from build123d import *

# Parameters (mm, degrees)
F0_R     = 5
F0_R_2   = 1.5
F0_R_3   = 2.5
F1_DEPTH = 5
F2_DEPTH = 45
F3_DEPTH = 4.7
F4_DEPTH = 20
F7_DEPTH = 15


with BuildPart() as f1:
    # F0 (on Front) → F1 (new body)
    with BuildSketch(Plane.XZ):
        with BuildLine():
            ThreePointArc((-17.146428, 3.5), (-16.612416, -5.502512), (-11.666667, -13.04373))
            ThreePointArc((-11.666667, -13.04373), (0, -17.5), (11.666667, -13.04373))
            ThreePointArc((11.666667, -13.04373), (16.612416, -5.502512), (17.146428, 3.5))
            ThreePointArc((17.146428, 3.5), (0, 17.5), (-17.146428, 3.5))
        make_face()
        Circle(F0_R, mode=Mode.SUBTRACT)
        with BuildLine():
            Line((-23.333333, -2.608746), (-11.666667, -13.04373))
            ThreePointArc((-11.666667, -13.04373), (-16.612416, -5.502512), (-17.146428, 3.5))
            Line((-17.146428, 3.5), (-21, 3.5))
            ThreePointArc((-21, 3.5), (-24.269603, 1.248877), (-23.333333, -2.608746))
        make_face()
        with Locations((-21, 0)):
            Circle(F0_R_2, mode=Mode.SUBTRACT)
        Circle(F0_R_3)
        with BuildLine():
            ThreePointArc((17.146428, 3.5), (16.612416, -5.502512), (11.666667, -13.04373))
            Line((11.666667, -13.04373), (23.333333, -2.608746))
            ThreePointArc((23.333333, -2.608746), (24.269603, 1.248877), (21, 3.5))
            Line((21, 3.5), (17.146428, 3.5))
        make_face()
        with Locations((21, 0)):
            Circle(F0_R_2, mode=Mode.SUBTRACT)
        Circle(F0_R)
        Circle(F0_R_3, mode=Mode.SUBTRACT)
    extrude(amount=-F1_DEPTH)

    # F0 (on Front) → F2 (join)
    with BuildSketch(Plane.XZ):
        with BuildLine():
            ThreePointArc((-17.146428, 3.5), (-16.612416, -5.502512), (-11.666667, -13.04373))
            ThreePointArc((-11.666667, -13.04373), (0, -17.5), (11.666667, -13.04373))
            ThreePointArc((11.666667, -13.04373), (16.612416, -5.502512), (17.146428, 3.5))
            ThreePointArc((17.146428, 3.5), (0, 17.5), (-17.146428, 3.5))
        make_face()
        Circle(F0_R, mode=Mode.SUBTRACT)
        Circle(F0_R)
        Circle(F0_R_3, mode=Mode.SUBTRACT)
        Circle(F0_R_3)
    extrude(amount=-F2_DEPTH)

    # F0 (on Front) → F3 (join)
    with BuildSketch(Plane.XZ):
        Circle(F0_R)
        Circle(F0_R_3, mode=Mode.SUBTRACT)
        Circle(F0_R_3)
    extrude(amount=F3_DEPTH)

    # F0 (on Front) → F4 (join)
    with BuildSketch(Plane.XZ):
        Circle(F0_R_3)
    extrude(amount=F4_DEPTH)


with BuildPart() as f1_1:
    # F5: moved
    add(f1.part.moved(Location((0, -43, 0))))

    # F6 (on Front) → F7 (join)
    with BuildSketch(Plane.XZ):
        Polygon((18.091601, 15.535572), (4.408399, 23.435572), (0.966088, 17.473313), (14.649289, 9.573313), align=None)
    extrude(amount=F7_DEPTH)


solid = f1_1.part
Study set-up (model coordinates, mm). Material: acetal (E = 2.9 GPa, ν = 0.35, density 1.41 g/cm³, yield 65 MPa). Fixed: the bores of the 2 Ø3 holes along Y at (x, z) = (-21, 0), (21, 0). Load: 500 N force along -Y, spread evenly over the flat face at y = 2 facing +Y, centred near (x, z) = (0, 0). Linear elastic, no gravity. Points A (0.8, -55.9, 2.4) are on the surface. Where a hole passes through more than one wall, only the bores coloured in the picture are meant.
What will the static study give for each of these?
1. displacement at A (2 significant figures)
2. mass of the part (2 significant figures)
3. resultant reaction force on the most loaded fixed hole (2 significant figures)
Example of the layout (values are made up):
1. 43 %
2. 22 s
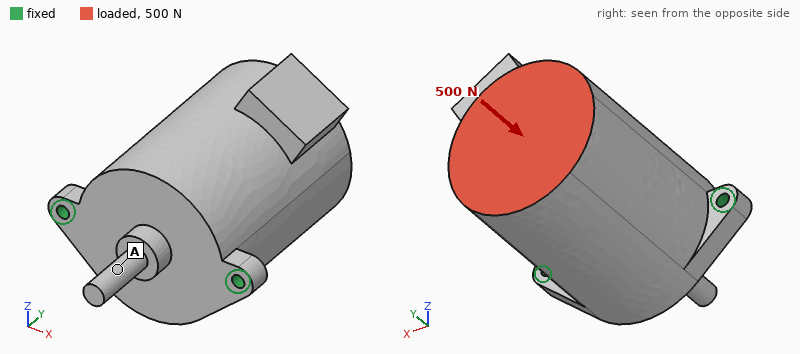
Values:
1. 0.063 mm
2. 65 g
3. 270 N
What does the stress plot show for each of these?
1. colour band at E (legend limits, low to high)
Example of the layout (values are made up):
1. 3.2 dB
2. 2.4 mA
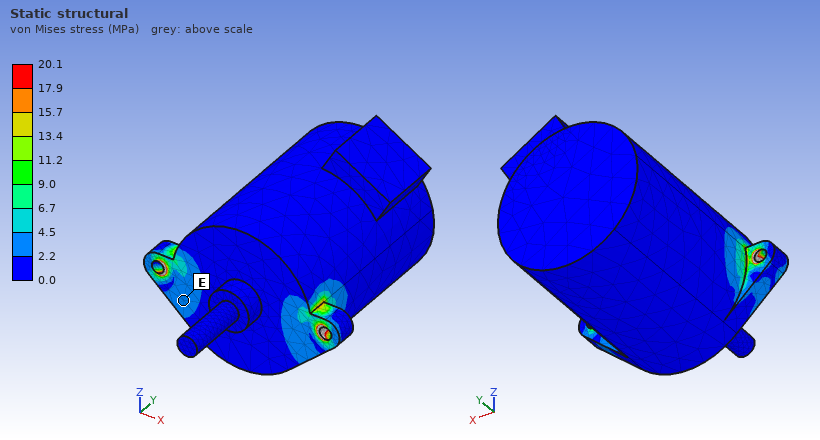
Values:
1. 2.2 to 4.5 MPa
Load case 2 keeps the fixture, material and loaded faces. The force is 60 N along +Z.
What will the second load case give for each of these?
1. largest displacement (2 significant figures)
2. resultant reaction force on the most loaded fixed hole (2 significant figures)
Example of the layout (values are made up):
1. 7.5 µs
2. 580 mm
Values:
1. 0.97 mm
2. 34 N
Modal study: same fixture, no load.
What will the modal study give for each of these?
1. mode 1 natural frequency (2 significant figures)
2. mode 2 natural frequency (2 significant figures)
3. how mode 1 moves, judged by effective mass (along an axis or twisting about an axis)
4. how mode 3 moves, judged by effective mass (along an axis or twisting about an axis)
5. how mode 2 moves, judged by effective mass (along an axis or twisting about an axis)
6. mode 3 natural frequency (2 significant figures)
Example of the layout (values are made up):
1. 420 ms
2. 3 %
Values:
1. 270 Hz
2. 1400 Hz
3. along Z
4. along Y
5. along X
6. 2000 Hz
